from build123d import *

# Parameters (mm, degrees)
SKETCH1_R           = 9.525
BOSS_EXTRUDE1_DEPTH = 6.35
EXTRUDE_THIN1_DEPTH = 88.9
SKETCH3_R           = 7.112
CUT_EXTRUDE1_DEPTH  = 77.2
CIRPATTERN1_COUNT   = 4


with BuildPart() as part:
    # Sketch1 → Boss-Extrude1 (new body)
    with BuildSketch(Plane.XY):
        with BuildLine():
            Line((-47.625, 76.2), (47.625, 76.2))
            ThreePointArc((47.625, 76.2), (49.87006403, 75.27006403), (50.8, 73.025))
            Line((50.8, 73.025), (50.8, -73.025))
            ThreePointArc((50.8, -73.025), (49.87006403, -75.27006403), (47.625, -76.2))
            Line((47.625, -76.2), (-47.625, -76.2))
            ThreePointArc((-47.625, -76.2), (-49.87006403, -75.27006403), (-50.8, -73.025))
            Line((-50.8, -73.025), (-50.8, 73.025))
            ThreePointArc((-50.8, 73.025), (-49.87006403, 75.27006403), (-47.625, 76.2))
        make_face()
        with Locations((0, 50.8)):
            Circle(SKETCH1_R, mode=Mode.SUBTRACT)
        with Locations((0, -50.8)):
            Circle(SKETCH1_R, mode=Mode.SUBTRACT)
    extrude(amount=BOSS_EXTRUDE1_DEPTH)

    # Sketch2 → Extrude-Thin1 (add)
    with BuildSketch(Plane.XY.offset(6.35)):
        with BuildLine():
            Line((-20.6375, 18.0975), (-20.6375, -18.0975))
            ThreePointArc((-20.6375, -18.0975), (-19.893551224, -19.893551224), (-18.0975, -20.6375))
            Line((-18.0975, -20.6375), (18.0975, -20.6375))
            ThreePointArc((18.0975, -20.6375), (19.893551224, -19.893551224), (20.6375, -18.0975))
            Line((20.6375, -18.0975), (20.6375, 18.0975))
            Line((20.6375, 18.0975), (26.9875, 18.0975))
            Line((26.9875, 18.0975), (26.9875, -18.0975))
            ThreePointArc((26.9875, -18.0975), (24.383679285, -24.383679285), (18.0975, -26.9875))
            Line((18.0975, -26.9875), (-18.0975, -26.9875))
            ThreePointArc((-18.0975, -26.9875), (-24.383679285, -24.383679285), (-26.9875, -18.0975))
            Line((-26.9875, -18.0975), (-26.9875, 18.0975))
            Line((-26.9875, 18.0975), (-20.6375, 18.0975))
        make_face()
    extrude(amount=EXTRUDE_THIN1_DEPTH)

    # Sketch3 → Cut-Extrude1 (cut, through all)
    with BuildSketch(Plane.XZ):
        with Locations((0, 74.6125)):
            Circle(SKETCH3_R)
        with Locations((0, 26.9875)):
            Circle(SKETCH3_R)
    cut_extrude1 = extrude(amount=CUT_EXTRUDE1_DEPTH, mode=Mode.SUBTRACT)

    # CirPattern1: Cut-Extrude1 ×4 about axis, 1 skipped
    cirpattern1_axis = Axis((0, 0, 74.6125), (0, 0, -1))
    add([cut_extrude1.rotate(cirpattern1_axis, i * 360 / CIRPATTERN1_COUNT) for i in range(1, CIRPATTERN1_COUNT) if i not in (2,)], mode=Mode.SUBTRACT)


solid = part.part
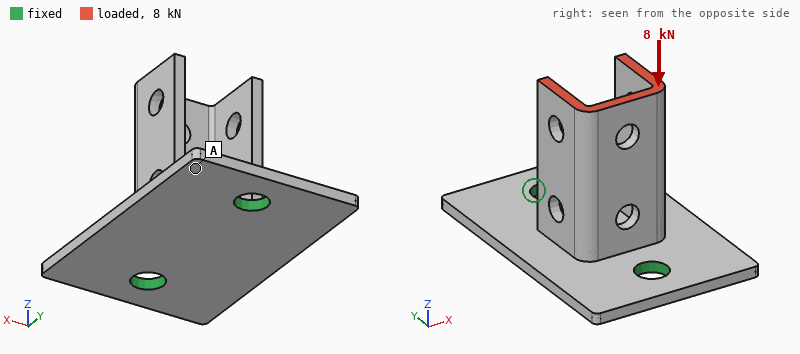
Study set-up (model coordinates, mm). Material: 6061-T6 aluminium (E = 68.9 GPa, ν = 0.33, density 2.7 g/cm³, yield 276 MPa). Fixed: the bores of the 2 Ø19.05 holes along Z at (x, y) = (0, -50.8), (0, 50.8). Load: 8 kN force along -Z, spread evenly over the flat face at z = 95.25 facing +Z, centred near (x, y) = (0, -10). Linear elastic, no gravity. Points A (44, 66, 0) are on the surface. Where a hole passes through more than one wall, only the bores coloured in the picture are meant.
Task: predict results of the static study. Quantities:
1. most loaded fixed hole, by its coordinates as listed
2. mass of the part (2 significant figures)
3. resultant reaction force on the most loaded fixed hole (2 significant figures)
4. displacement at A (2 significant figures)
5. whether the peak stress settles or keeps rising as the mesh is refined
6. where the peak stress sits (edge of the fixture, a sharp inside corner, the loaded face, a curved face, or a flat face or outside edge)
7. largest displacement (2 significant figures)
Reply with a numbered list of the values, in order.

1. (0, -50.8)
2. 430 g
3. 5.2 kN
4. 0.028 mm
5. keeps rising
6. edge of the fixture
7. 0.18 mm
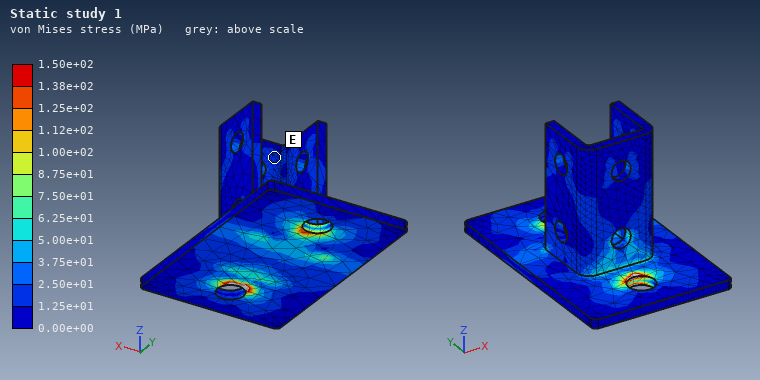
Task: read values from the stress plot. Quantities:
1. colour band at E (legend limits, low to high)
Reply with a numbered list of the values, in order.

1. 1.25e+01 to 2.50e+01 MPa
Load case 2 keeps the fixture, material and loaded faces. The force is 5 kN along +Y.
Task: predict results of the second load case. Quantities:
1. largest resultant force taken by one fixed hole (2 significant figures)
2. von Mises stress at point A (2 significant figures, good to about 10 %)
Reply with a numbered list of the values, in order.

1. 6.8 kN
2. 14 MPa
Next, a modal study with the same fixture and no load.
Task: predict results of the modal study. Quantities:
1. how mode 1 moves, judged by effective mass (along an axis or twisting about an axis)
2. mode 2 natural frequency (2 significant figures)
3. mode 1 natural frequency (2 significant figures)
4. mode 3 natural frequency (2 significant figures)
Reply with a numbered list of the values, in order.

1. along X
2. 1600 Hz
3. 860 Hz
4. 2000 Hz
